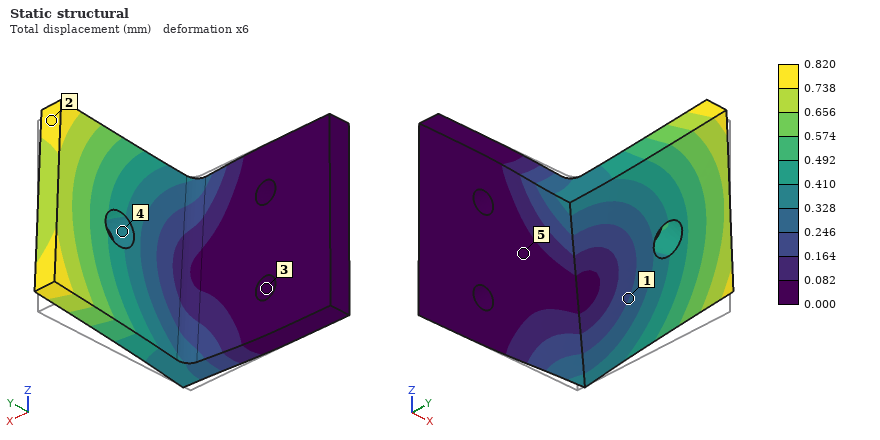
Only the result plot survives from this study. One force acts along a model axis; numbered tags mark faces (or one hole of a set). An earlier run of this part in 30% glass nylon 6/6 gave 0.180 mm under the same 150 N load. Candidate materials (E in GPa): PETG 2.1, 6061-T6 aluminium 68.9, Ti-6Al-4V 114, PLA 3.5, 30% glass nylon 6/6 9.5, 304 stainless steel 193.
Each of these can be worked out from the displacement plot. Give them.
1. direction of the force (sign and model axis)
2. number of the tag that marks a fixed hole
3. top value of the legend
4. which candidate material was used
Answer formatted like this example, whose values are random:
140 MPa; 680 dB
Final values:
+Z; 3; 0.820 mm; PETG
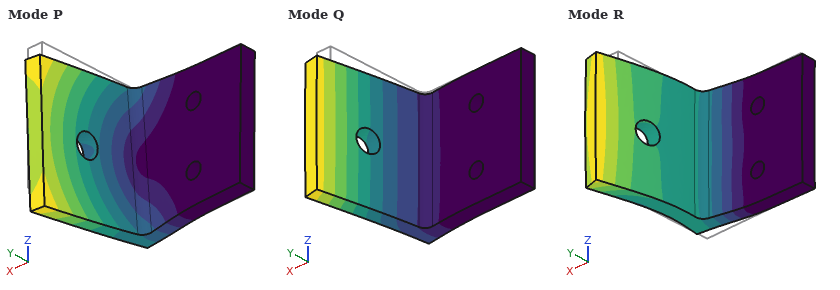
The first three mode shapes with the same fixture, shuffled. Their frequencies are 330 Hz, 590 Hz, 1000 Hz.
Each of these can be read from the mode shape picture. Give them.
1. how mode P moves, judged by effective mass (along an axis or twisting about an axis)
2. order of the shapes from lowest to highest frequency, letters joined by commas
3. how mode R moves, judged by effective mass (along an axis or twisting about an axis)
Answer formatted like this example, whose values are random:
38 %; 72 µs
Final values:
along Z; Q, P, R; along Y
